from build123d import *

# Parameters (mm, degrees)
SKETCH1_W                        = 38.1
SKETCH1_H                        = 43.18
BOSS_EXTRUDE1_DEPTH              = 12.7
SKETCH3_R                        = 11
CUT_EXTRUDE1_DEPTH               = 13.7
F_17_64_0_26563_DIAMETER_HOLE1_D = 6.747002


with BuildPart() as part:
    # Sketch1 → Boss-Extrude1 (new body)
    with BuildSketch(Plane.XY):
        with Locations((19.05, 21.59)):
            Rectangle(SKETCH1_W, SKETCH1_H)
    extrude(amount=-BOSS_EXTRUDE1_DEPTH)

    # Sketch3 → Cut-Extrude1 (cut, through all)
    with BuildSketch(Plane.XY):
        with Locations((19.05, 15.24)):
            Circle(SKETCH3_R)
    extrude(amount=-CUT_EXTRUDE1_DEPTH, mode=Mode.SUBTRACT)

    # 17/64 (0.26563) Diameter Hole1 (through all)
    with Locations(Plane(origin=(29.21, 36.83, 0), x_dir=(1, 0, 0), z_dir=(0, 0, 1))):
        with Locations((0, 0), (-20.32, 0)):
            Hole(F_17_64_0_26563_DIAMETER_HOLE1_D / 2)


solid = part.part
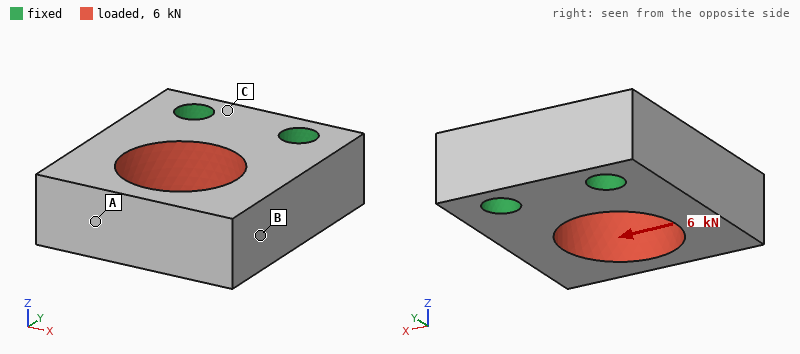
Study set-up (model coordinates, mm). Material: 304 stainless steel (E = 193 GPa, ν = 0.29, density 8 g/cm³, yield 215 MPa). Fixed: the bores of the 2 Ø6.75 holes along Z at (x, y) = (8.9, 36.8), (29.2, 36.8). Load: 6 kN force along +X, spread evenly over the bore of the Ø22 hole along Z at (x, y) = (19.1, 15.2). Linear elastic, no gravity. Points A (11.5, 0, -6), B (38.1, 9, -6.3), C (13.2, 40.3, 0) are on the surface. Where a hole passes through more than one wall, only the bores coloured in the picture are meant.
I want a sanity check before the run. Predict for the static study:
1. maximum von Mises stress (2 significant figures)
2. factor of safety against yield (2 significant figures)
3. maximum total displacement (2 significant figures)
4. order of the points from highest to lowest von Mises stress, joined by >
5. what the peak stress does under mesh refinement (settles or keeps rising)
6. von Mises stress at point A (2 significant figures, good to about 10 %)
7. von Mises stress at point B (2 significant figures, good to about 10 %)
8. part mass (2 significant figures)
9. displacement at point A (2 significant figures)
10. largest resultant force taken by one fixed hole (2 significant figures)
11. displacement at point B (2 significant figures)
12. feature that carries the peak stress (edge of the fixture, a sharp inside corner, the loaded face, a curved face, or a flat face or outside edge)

100 MPa
2.1
29 µm
A > B > C
settles
56 MPa
26 MPa
120 g
27 µm
5.0 kN
22 µm
the loaded face
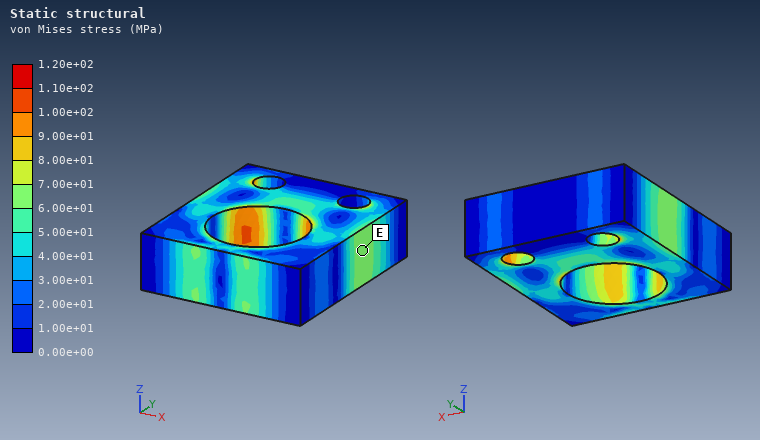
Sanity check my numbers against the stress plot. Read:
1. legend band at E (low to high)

6.00e+01 to 7.00e+01 MPa
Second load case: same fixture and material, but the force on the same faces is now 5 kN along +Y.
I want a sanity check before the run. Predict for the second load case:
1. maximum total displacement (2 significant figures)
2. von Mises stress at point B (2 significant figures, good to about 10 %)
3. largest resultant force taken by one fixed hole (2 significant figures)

6.3 µm
9.9 MPa
2.5 kN
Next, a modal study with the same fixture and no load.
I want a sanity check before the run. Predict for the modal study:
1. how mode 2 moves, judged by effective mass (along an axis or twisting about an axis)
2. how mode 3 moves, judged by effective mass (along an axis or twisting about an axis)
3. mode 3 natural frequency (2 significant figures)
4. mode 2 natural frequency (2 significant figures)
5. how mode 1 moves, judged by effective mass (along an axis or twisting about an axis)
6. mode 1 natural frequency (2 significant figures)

along X
twisting about Y
11 kHz
9300 Hz
along Z
6800 Hz
